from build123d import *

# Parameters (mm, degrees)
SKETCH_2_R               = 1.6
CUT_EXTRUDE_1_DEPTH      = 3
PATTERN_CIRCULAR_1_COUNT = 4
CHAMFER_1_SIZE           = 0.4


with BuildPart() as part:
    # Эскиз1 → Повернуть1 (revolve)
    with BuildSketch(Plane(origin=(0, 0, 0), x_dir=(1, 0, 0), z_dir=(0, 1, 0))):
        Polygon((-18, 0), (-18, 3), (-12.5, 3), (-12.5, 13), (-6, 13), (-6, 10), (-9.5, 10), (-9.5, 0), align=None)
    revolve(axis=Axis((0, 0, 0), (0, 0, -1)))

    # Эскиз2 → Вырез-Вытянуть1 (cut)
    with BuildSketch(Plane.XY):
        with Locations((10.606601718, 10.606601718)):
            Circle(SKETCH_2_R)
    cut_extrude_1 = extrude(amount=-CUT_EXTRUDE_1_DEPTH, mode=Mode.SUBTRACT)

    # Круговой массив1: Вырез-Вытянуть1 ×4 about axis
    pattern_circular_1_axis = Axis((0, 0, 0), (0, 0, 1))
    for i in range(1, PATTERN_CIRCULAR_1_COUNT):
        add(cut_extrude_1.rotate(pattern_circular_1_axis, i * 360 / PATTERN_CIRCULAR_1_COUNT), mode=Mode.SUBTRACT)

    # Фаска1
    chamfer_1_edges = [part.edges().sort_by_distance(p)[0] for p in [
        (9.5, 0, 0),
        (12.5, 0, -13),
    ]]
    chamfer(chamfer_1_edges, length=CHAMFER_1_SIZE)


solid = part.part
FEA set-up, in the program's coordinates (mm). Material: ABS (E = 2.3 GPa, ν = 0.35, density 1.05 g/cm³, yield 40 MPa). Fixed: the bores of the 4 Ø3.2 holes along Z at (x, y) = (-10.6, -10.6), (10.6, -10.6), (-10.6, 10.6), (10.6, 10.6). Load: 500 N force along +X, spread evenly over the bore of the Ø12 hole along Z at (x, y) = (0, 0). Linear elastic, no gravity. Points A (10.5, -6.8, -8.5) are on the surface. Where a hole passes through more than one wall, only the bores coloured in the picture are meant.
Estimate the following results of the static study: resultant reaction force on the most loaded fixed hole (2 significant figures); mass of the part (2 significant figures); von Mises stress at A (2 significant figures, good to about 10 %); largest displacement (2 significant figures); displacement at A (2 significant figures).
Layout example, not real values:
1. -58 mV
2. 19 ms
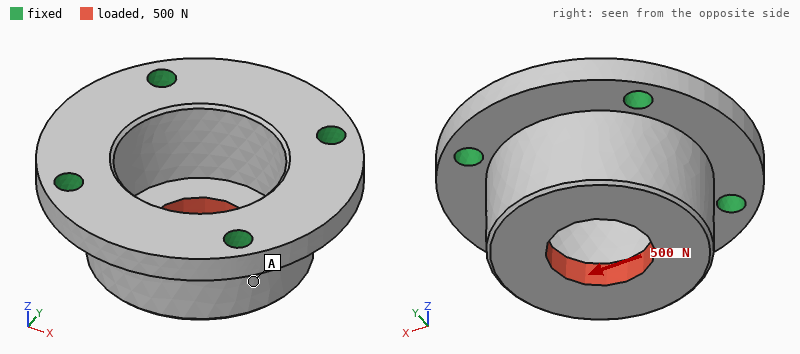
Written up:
1. 180 N
2. 4.9 g
3. 2.9 MPa
4. 0.13 mm
5. 0.077 mm
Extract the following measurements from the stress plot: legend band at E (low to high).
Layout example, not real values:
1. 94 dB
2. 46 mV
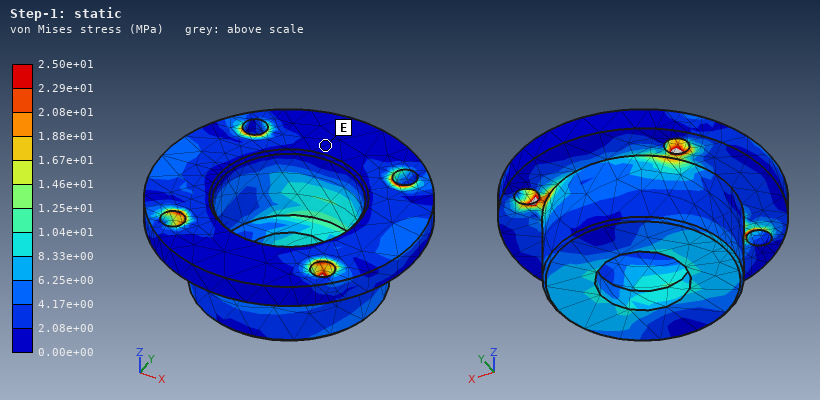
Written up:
1. 0.00e+00 to 2.08e+00 MPa
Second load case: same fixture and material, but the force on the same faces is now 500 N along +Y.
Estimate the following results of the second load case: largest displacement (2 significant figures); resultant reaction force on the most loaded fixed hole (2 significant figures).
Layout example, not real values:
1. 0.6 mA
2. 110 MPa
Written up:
1. 0.13 mm
2. 180 N
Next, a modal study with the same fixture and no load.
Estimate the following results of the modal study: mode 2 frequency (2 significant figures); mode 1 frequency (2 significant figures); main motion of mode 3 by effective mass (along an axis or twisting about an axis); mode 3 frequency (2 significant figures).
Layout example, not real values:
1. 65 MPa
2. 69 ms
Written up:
1. 7900 Hz
2. 7900 Hz
3. along Z
4. 9400 Hz
